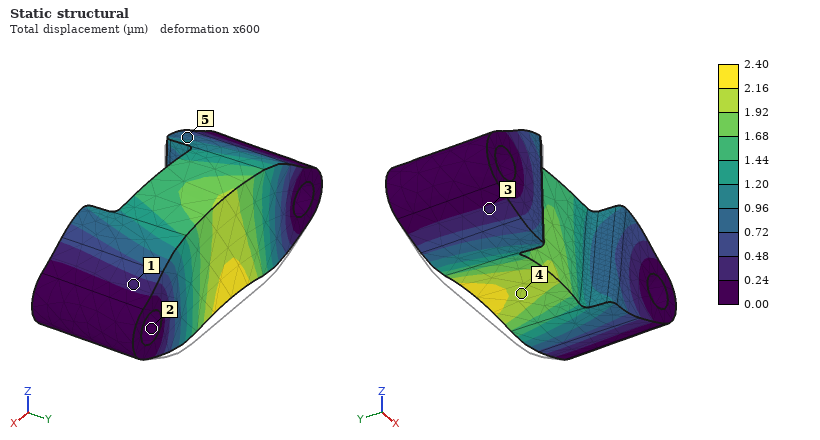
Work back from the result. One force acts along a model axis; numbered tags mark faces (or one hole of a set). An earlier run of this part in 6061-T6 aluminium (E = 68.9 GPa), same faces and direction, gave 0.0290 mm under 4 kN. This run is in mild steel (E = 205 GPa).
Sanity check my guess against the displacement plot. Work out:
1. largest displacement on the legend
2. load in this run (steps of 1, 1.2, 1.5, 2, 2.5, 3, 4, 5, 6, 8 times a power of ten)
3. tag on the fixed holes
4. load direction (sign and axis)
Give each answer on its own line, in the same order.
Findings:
2.40 µm
1 kN
2
+Z
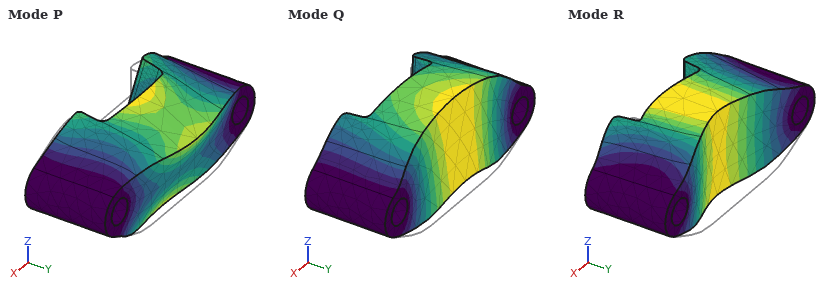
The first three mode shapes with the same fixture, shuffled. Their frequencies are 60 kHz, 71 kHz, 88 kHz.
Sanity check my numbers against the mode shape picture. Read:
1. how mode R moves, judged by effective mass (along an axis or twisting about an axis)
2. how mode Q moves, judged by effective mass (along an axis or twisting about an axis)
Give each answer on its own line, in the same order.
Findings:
along Y
along Z
